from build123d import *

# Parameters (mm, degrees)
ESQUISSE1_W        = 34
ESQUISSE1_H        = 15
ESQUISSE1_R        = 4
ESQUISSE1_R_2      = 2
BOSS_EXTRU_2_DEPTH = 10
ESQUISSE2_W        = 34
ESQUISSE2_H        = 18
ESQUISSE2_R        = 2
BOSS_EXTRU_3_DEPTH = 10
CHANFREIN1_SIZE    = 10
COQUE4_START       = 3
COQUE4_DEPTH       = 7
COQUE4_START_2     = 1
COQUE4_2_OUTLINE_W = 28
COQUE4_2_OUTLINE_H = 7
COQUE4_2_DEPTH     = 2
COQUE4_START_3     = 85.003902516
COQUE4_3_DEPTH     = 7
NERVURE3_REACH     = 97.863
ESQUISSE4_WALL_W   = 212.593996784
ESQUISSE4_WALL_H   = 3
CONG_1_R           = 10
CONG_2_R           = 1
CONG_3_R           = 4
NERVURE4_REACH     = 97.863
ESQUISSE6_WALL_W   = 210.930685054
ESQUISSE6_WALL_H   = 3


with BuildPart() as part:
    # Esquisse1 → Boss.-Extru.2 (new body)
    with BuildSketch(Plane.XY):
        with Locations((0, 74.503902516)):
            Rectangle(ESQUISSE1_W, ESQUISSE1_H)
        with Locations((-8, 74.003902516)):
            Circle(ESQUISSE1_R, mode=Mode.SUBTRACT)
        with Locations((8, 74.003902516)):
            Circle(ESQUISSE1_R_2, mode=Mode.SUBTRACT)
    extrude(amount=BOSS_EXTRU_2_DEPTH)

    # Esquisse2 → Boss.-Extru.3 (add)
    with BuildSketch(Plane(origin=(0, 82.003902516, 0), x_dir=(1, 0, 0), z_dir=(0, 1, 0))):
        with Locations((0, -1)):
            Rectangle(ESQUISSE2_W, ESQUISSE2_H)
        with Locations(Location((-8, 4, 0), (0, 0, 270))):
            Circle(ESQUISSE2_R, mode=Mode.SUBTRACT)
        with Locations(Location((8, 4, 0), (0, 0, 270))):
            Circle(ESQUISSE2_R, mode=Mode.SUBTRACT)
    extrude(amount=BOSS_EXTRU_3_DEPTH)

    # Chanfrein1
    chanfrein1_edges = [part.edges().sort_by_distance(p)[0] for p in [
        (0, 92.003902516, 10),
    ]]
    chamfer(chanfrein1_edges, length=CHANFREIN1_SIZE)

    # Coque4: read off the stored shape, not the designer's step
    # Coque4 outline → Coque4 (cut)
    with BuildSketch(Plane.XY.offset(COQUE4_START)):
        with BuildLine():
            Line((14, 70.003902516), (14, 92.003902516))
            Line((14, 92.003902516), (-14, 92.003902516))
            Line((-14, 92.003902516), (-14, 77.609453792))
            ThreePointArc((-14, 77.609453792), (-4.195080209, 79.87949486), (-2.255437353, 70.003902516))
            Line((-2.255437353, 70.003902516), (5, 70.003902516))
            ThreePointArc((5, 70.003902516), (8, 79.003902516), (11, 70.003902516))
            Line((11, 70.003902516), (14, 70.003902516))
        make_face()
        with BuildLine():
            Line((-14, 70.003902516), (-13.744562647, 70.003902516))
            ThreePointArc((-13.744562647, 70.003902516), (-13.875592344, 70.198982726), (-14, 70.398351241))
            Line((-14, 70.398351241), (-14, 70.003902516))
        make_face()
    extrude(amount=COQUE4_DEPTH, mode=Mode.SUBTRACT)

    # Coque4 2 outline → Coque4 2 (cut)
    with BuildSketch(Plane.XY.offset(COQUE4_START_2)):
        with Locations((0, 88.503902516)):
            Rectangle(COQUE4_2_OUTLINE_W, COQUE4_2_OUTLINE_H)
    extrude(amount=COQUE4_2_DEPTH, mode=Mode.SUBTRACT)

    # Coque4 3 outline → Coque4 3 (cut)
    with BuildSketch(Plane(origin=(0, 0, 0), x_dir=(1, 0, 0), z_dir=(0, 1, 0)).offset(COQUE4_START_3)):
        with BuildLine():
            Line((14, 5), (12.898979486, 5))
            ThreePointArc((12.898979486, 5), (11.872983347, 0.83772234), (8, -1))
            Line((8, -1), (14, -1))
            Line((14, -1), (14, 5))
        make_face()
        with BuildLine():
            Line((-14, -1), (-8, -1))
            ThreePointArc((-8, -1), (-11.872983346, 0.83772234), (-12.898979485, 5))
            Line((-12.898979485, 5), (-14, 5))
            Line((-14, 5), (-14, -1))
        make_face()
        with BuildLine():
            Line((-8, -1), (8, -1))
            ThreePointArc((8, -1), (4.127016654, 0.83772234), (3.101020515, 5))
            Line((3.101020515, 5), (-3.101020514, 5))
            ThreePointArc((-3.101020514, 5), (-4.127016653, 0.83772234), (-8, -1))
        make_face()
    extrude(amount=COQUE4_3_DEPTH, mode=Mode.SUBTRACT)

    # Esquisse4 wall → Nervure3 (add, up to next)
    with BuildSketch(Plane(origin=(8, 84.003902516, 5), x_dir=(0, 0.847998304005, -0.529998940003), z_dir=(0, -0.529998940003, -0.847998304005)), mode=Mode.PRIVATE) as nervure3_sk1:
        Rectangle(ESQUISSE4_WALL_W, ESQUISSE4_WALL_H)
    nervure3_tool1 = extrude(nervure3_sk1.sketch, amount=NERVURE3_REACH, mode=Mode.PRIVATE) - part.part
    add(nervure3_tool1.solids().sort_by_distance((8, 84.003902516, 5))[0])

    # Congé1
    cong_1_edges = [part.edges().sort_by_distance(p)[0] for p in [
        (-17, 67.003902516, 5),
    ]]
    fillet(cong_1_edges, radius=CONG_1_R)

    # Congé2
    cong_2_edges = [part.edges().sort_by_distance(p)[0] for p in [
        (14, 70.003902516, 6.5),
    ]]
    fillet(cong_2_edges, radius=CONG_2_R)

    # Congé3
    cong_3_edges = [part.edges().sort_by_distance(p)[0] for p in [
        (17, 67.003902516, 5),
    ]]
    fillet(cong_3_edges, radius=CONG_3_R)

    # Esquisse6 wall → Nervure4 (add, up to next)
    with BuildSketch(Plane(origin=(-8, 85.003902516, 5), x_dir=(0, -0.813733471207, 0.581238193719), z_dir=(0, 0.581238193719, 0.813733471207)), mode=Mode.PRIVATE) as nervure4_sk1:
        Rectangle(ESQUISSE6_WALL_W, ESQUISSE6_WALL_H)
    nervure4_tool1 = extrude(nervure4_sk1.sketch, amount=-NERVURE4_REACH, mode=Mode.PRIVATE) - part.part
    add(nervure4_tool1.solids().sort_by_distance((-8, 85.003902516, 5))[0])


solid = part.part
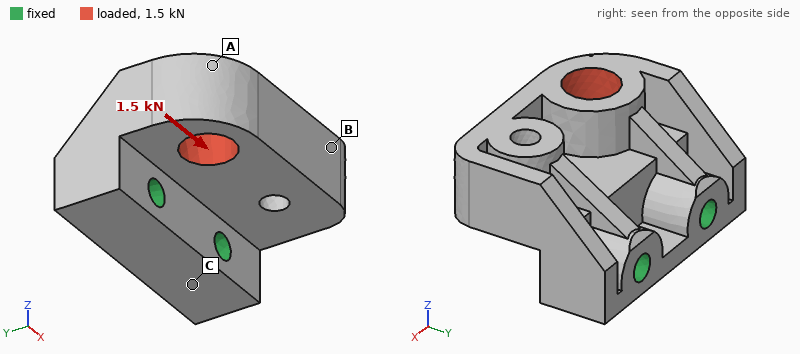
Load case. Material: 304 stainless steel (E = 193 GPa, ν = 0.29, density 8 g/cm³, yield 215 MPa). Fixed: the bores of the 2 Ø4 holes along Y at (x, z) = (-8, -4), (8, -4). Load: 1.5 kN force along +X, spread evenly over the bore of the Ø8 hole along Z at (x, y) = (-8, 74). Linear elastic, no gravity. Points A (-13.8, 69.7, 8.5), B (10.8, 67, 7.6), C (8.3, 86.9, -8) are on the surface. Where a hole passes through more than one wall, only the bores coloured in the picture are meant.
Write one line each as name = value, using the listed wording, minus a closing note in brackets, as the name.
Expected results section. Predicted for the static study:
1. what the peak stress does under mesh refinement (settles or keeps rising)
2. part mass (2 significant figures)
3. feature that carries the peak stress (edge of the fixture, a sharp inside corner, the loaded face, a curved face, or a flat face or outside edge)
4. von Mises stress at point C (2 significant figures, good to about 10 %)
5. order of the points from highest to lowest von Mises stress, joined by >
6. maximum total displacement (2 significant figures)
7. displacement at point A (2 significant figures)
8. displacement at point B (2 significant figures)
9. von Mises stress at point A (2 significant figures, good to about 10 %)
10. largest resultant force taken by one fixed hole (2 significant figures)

what the peak stress does under mesh refinement = keeps rising
part mass = 49 g
feature that carries the peak stress = edge of the fixture
von Mises stress at point C = 9.8 MPa
order of the points from highest to lowest von Mises stress, joined by > = A > C > B
maximum total displacement = 8.2 µm
displacement at point A = 7.9 µm
displacement at point B = 6.4 µm
von Mises stress at point A = 17 MPa
largest resultant force taken by one fixed hole = 1.2 kN
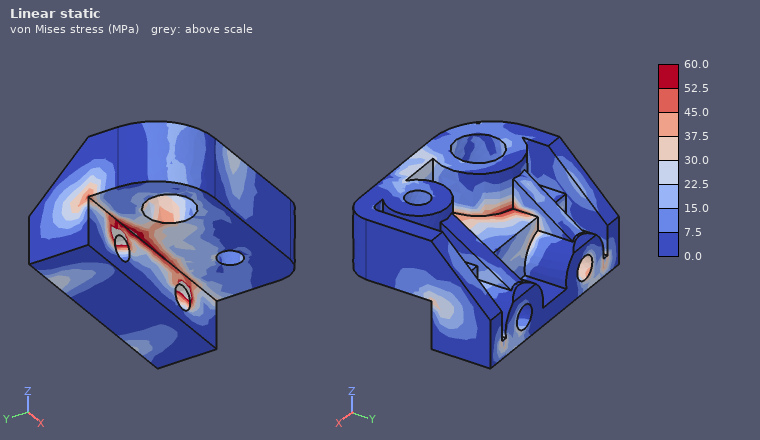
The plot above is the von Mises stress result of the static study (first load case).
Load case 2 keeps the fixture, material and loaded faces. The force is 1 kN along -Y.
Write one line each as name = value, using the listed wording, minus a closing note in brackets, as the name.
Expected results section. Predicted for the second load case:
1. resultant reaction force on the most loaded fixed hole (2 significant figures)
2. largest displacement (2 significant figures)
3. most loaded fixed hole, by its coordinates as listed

resultant reaction force on the most loaded fixed hole = 900 N
largest displacement = 14 µm
most loaded fixed hole, by its coordinates as listed = (-8, -4)
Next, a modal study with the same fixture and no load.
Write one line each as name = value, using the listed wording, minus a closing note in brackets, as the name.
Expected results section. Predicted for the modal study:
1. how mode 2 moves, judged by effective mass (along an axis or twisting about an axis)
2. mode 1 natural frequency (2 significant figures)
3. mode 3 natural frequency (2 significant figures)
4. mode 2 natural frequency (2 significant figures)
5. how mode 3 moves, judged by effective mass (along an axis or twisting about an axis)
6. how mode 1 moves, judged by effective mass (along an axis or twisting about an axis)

how mode 2 moves, judged by effective mass = twisting about Y
mode 1 natural frequency = 7600 Hz
mode 3 natural frequency = 16 kHz
mode 2 natural frequency = 12 kHz
how mode 3 moves, judged by effective mass = along X
how mode 1 moves, judged by effective mass = along Z
